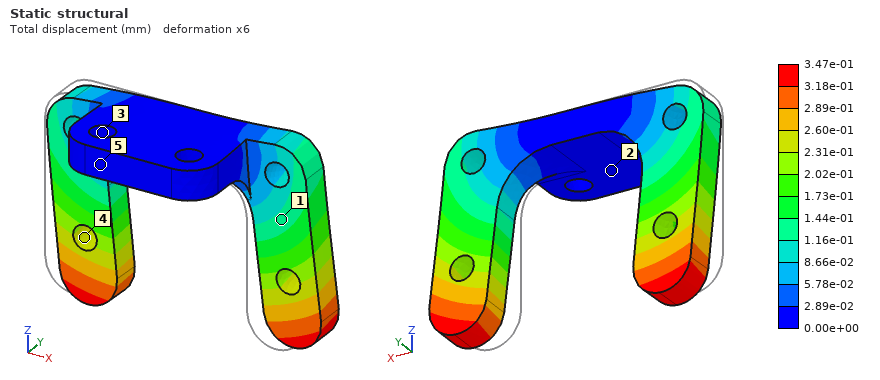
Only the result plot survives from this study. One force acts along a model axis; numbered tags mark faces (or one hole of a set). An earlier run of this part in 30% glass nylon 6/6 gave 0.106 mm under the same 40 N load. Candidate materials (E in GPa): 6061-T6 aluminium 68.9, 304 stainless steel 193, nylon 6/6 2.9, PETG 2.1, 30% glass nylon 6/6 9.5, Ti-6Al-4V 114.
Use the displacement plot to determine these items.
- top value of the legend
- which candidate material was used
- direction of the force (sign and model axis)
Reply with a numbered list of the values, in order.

1. 3.47e-01 mm
2. nylon 6/6
3. +X
